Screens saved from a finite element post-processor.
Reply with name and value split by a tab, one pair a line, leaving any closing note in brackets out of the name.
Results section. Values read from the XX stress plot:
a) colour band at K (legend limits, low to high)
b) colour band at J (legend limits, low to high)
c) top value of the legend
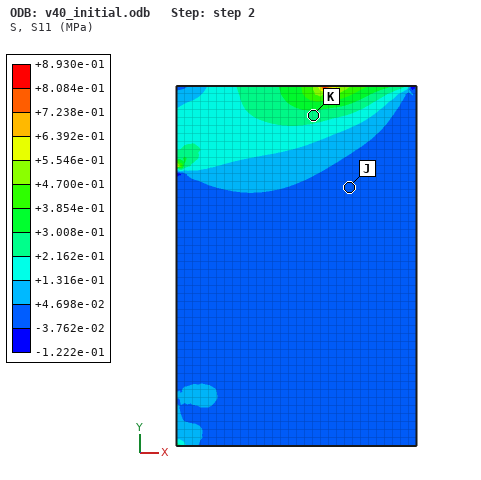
colour band at K	+2.162e-01 to +3.008e-01 MPa
colour band at J	-3.762e-02 to +4.698e-02 MPa
top value of the legend	+8.930e-01 MPa
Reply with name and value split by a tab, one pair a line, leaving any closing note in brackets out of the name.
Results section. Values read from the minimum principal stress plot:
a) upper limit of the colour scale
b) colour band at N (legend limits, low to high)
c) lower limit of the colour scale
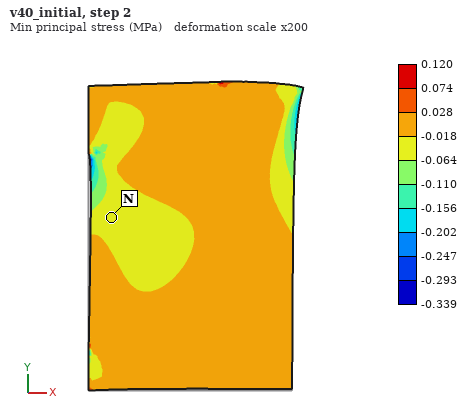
upper limit of the colour scale	0.120 MPa
colour band at N	-0.064 to -0.018 MPa
lower limit of the colour scale	-0.339 MPa
